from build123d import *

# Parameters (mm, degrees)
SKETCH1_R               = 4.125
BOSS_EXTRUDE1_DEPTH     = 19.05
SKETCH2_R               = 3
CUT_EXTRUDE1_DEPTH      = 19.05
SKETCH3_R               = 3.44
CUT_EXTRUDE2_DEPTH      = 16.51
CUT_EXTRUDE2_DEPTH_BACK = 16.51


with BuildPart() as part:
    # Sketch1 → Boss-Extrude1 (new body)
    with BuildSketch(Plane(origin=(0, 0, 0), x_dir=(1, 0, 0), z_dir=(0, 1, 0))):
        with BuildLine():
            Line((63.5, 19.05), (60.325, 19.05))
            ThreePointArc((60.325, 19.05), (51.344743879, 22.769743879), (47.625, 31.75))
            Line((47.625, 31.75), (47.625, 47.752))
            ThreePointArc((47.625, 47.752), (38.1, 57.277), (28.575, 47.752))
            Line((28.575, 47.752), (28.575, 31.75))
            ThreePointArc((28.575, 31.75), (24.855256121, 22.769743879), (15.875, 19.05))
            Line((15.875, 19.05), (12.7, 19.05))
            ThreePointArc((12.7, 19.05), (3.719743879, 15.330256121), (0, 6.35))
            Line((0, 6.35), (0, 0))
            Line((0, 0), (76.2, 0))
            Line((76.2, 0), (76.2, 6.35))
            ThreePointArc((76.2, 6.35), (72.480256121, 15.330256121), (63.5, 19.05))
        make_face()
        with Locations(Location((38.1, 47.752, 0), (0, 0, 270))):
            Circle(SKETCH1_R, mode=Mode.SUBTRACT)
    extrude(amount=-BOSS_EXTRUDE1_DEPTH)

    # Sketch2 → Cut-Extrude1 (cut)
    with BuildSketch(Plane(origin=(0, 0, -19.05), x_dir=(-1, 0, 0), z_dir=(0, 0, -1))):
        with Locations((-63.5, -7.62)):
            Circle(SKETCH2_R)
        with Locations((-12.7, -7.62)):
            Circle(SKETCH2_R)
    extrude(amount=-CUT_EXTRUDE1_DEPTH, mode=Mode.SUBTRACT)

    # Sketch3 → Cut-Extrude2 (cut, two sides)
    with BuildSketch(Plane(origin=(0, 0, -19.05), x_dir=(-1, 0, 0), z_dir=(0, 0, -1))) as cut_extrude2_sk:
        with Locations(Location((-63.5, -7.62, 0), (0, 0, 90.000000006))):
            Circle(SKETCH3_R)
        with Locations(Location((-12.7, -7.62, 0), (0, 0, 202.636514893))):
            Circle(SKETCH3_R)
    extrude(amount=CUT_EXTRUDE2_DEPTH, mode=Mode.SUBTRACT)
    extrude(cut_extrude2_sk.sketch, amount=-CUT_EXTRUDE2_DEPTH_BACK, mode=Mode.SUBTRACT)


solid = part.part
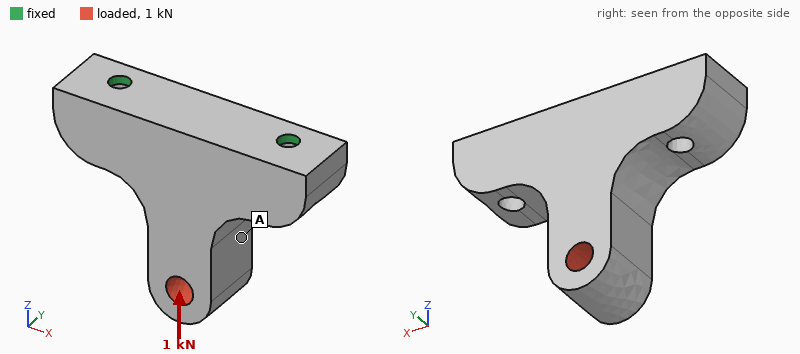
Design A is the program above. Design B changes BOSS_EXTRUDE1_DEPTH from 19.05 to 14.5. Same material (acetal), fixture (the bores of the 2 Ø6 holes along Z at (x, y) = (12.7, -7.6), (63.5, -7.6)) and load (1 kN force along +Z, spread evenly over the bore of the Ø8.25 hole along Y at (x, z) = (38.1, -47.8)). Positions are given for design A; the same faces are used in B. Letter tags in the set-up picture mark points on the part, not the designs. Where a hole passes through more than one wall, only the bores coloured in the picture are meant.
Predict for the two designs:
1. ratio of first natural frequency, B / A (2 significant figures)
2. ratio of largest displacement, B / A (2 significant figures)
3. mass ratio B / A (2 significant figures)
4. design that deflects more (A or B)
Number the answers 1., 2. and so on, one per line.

1. 1.1
2. 0.44
3. 0.75
4. A
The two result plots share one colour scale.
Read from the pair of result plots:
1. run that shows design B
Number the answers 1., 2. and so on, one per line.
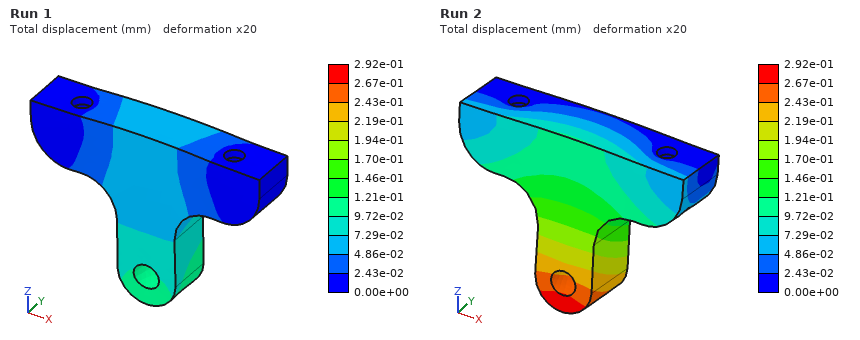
1. Run 1
